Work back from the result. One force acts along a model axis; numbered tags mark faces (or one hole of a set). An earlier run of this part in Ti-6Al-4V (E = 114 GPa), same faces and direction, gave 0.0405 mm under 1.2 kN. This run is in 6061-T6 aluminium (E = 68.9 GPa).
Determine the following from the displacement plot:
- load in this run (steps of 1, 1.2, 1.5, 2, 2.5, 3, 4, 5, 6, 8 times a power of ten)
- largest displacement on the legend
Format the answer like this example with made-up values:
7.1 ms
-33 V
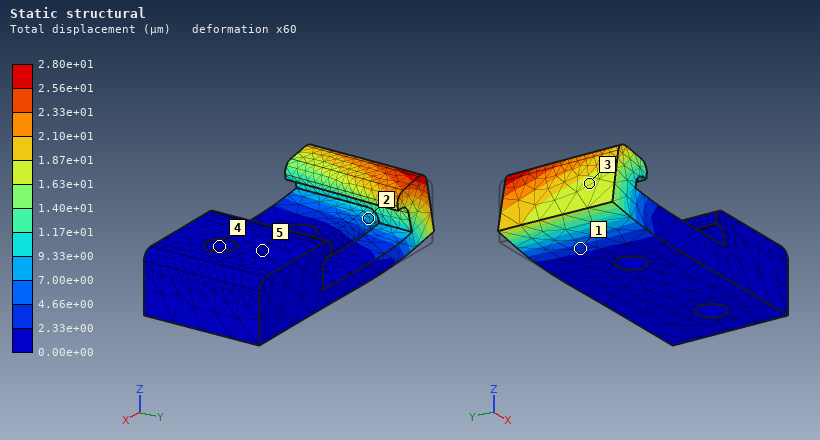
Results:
500 N
2.80e+01 µm
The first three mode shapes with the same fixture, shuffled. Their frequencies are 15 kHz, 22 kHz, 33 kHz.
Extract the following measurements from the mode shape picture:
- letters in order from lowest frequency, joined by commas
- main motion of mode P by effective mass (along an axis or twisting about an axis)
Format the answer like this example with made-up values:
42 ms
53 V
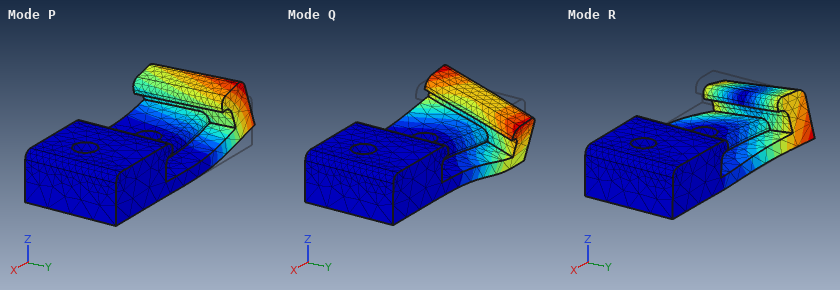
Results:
P, Q, R
along Z
